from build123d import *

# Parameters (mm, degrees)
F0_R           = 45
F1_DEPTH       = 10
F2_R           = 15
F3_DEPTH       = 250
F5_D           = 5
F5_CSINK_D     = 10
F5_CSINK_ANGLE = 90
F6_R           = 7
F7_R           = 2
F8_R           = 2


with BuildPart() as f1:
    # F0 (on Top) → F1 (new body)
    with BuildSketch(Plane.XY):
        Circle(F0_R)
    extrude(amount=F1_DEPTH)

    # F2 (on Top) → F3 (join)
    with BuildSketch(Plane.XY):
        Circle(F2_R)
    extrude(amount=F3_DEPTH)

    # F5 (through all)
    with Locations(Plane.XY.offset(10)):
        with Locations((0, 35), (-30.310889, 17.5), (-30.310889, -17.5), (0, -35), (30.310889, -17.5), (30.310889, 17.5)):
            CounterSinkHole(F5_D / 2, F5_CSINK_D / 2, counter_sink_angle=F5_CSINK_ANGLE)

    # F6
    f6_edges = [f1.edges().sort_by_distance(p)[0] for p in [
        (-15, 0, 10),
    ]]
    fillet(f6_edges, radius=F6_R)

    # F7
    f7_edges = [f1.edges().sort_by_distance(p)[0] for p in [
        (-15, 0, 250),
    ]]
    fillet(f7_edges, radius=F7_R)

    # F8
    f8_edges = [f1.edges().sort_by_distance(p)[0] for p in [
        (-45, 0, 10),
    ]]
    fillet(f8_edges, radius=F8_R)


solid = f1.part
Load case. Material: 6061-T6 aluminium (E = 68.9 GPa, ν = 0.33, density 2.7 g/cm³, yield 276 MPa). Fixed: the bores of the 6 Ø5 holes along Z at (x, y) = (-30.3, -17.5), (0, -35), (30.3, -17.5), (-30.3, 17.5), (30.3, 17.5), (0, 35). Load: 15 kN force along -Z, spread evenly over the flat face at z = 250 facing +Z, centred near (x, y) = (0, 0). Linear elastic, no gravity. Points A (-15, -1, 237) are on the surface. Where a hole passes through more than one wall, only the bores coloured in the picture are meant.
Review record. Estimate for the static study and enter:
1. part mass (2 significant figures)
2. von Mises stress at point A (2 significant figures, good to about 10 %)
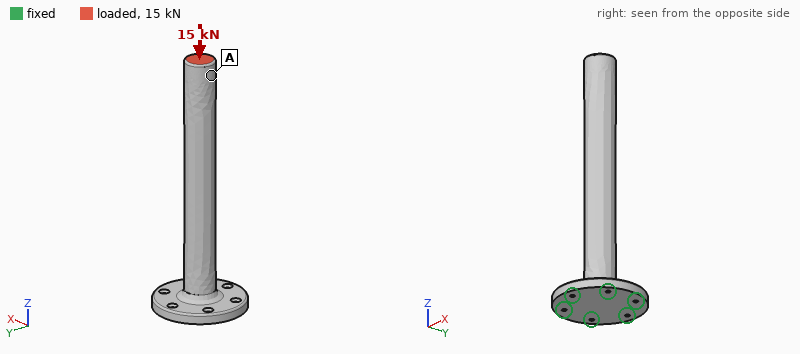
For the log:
630 g
20 MPa
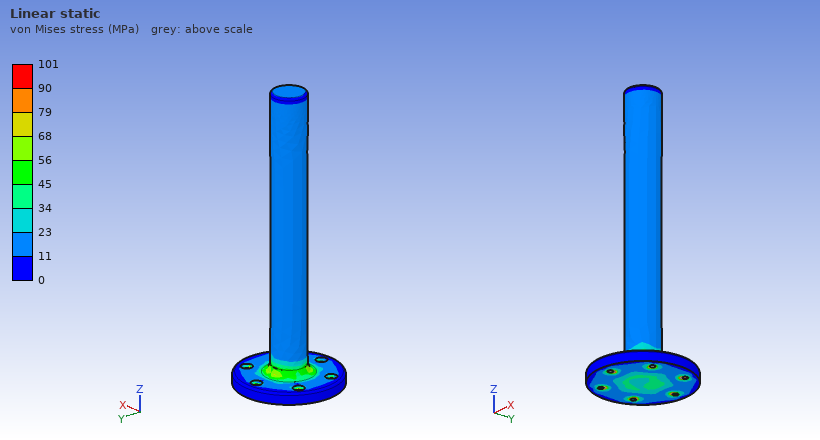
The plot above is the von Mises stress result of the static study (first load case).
